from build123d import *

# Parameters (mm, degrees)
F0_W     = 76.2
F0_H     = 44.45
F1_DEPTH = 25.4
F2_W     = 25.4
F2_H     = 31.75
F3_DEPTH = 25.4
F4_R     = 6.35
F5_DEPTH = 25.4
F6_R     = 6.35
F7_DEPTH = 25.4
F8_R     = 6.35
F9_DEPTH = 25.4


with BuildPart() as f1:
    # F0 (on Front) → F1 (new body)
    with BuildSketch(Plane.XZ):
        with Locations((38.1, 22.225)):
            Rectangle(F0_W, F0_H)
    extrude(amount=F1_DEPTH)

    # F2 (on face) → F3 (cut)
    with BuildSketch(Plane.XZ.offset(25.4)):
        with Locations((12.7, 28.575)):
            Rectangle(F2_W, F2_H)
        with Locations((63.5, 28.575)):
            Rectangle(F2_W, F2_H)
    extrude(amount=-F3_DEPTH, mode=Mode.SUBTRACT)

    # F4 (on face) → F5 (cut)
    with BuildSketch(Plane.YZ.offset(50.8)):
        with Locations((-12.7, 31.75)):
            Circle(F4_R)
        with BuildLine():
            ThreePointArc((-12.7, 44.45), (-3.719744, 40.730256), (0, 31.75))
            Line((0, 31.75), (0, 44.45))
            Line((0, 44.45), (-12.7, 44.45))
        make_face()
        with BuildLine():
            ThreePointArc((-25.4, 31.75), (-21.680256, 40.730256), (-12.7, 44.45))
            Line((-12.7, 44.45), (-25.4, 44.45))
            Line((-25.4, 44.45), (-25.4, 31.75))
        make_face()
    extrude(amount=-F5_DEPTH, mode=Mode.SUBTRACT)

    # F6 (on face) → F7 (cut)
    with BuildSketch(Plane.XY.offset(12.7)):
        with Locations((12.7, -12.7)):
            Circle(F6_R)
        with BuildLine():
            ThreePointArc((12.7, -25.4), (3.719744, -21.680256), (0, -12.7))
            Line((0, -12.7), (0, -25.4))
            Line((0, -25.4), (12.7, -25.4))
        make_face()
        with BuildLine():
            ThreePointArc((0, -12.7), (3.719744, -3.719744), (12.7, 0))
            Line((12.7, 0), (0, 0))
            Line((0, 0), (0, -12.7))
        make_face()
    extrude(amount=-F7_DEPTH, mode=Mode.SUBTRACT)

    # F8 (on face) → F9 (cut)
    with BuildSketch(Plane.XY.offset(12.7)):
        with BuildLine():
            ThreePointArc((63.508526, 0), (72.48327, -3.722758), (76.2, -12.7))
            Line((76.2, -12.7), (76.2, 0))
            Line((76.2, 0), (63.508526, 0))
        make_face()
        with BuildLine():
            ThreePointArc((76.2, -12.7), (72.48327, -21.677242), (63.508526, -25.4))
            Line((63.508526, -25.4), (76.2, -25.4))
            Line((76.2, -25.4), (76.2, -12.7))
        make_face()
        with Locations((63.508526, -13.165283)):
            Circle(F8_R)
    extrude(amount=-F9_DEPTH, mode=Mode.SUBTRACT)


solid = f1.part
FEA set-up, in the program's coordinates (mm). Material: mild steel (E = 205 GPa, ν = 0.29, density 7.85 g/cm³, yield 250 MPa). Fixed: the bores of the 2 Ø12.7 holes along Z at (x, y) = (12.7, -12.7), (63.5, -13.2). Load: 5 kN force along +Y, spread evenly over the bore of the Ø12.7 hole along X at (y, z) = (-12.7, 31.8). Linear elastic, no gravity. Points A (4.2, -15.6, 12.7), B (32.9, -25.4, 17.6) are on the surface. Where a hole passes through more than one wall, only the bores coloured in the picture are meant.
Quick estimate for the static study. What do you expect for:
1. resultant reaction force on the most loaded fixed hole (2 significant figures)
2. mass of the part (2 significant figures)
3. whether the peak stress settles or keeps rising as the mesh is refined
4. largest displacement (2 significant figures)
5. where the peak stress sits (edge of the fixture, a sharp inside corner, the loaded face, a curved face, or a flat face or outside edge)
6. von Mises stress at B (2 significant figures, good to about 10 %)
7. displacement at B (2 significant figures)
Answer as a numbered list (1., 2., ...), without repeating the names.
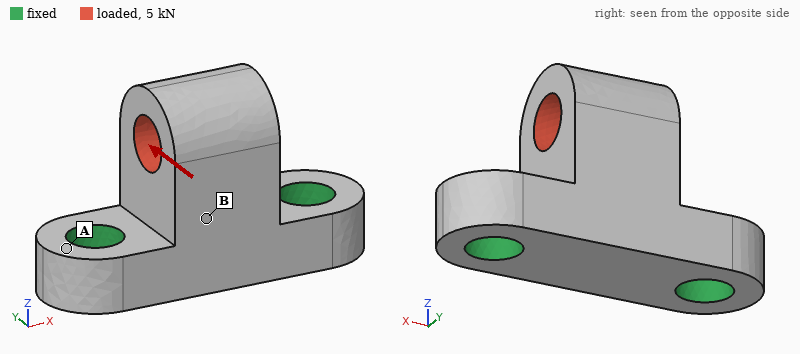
1. 2.5 kN
2. 280 g
3. keeps rising
4. 37 µm
5. edge of the fixture
6. 27 MPa
7. 14 µm
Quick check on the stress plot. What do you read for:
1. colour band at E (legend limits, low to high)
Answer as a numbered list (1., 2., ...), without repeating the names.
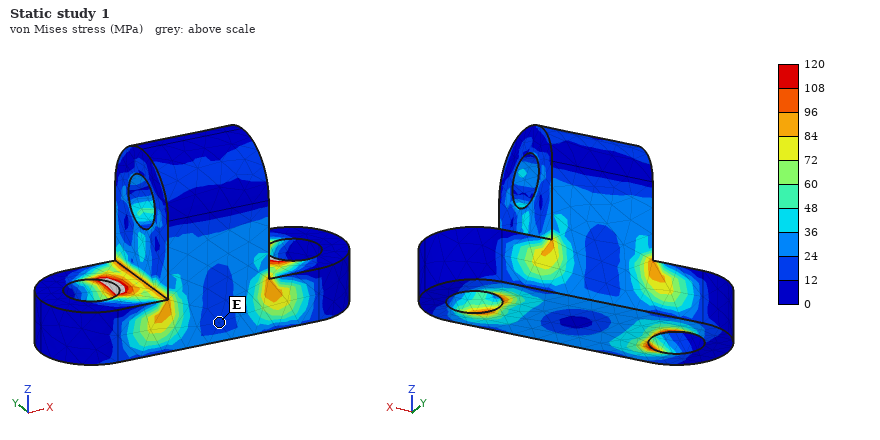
1. 12 to 24 MPa
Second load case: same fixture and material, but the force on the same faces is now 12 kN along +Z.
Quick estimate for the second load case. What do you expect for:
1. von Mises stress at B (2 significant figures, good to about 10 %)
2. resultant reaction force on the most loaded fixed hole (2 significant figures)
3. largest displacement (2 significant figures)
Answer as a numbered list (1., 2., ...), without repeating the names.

1. 20 MPa
2. 6.2 kN
3. 9.2 µm
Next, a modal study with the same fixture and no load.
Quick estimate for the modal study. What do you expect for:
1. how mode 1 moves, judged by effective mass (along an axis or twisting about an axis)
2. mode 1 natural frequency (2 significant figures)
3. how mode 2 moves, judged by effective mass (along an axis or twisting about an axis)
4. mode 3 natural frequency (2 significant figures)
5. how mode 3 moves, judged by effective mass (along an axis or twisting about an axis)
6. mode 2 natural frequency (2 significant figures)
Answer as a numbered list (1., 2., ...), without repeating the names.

1. along Y
2. 7100 Hz
3. along X
4. 17 kHz
5. along Z
6. 12 kHz
